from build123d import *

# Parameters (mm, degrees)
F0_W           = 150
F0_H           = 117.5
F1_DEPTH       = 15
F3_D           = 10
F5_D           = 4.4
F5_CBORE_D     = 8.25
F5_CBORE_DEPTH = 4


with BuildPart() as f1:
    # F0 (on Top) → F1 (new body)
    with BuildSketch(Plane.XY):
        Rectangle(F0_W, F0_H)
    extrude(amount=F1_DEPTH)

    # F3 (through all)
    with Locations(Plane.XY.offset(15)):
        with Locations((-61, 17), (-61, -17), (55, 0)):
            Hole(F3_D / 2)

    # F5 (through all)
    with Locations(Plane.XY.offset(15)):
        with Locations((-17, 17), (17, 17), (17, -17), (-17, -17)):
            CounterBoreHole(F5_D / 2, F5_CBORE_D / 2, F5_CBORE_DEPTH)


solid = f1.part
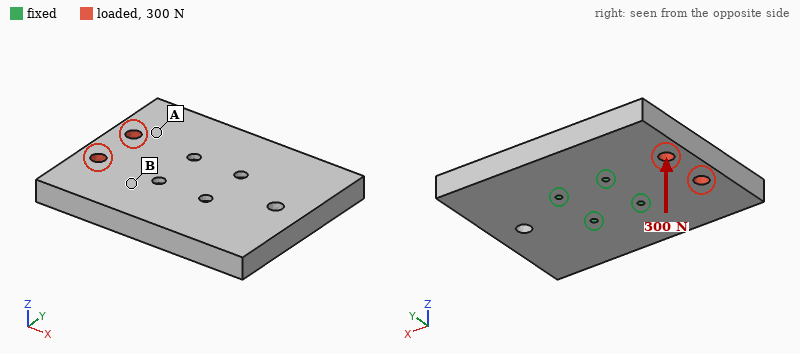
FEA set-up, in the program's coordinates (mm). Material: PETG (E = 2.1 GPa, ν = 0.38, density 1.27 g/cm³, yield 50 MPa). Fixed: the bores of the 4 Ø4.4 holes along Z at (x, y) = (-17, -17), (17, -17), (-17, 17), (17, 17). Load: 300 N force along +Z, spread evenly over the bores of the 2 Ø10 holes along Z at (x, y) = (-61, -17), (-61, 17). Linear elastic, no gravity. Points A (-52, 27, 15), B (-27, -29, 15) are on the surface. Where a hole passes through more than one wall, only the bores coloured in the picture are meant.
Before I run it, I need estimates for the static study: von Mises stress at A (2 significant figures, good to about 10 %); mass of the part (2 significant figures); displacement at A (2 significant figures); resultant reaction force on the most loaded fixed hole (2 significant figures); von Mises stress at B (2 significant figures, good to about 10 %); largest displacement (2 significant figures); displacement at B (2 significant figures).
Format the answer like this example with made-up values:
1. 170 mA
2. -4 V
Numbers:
1. 1.00 MPa
2. 330 g
3. 0.18 mm
4. 280 N
5. 2.2 MPa
6. 0.34 mm
7. 0.054 mm
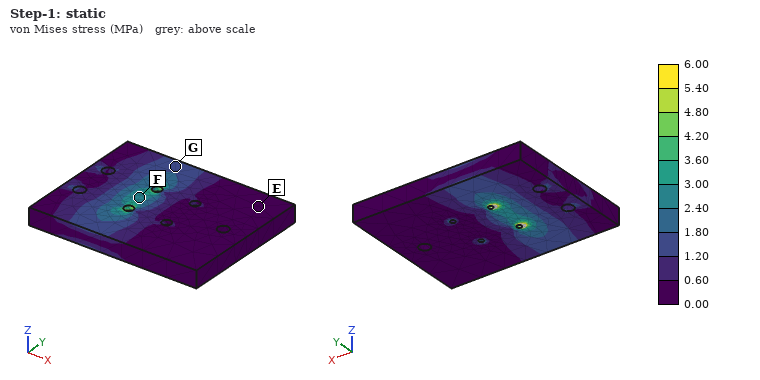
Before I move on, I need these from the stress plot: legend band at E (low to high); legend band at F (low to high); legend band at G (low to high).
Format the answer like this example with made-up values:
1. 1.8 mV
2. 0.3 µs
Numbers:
1. 0.00 to 0.60 MPa
2. 2.40 to 3.00 MPa
3. 1.20 to 1.80 MPa
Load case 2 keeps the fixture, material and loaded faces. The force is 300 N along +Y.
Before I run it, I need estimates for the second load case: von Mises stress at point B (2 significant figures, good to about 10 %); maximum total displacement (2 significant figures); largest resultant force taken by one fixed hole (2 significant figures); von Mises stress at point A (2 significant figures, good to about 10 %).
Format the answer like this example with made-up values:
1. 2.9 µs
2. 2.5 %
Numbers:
1. 0.29 MPa
2. 39 µm
3. 250 N
4. 0.29 MPa
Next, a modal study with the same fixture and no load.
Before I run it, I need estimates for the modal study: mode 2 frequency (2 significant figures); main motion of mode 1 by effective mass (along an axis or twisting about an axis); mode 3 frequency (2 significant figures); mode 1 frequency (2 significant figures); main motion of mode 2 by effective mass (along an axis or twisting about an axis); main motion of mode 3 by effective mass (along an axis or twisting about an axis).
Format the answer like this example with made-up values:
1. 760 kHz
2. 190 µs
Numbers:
1. 700 Hz
2. twisting about Y
3. 800 Hz
4. 640 Hz
5. along Z
6. twisting about X
